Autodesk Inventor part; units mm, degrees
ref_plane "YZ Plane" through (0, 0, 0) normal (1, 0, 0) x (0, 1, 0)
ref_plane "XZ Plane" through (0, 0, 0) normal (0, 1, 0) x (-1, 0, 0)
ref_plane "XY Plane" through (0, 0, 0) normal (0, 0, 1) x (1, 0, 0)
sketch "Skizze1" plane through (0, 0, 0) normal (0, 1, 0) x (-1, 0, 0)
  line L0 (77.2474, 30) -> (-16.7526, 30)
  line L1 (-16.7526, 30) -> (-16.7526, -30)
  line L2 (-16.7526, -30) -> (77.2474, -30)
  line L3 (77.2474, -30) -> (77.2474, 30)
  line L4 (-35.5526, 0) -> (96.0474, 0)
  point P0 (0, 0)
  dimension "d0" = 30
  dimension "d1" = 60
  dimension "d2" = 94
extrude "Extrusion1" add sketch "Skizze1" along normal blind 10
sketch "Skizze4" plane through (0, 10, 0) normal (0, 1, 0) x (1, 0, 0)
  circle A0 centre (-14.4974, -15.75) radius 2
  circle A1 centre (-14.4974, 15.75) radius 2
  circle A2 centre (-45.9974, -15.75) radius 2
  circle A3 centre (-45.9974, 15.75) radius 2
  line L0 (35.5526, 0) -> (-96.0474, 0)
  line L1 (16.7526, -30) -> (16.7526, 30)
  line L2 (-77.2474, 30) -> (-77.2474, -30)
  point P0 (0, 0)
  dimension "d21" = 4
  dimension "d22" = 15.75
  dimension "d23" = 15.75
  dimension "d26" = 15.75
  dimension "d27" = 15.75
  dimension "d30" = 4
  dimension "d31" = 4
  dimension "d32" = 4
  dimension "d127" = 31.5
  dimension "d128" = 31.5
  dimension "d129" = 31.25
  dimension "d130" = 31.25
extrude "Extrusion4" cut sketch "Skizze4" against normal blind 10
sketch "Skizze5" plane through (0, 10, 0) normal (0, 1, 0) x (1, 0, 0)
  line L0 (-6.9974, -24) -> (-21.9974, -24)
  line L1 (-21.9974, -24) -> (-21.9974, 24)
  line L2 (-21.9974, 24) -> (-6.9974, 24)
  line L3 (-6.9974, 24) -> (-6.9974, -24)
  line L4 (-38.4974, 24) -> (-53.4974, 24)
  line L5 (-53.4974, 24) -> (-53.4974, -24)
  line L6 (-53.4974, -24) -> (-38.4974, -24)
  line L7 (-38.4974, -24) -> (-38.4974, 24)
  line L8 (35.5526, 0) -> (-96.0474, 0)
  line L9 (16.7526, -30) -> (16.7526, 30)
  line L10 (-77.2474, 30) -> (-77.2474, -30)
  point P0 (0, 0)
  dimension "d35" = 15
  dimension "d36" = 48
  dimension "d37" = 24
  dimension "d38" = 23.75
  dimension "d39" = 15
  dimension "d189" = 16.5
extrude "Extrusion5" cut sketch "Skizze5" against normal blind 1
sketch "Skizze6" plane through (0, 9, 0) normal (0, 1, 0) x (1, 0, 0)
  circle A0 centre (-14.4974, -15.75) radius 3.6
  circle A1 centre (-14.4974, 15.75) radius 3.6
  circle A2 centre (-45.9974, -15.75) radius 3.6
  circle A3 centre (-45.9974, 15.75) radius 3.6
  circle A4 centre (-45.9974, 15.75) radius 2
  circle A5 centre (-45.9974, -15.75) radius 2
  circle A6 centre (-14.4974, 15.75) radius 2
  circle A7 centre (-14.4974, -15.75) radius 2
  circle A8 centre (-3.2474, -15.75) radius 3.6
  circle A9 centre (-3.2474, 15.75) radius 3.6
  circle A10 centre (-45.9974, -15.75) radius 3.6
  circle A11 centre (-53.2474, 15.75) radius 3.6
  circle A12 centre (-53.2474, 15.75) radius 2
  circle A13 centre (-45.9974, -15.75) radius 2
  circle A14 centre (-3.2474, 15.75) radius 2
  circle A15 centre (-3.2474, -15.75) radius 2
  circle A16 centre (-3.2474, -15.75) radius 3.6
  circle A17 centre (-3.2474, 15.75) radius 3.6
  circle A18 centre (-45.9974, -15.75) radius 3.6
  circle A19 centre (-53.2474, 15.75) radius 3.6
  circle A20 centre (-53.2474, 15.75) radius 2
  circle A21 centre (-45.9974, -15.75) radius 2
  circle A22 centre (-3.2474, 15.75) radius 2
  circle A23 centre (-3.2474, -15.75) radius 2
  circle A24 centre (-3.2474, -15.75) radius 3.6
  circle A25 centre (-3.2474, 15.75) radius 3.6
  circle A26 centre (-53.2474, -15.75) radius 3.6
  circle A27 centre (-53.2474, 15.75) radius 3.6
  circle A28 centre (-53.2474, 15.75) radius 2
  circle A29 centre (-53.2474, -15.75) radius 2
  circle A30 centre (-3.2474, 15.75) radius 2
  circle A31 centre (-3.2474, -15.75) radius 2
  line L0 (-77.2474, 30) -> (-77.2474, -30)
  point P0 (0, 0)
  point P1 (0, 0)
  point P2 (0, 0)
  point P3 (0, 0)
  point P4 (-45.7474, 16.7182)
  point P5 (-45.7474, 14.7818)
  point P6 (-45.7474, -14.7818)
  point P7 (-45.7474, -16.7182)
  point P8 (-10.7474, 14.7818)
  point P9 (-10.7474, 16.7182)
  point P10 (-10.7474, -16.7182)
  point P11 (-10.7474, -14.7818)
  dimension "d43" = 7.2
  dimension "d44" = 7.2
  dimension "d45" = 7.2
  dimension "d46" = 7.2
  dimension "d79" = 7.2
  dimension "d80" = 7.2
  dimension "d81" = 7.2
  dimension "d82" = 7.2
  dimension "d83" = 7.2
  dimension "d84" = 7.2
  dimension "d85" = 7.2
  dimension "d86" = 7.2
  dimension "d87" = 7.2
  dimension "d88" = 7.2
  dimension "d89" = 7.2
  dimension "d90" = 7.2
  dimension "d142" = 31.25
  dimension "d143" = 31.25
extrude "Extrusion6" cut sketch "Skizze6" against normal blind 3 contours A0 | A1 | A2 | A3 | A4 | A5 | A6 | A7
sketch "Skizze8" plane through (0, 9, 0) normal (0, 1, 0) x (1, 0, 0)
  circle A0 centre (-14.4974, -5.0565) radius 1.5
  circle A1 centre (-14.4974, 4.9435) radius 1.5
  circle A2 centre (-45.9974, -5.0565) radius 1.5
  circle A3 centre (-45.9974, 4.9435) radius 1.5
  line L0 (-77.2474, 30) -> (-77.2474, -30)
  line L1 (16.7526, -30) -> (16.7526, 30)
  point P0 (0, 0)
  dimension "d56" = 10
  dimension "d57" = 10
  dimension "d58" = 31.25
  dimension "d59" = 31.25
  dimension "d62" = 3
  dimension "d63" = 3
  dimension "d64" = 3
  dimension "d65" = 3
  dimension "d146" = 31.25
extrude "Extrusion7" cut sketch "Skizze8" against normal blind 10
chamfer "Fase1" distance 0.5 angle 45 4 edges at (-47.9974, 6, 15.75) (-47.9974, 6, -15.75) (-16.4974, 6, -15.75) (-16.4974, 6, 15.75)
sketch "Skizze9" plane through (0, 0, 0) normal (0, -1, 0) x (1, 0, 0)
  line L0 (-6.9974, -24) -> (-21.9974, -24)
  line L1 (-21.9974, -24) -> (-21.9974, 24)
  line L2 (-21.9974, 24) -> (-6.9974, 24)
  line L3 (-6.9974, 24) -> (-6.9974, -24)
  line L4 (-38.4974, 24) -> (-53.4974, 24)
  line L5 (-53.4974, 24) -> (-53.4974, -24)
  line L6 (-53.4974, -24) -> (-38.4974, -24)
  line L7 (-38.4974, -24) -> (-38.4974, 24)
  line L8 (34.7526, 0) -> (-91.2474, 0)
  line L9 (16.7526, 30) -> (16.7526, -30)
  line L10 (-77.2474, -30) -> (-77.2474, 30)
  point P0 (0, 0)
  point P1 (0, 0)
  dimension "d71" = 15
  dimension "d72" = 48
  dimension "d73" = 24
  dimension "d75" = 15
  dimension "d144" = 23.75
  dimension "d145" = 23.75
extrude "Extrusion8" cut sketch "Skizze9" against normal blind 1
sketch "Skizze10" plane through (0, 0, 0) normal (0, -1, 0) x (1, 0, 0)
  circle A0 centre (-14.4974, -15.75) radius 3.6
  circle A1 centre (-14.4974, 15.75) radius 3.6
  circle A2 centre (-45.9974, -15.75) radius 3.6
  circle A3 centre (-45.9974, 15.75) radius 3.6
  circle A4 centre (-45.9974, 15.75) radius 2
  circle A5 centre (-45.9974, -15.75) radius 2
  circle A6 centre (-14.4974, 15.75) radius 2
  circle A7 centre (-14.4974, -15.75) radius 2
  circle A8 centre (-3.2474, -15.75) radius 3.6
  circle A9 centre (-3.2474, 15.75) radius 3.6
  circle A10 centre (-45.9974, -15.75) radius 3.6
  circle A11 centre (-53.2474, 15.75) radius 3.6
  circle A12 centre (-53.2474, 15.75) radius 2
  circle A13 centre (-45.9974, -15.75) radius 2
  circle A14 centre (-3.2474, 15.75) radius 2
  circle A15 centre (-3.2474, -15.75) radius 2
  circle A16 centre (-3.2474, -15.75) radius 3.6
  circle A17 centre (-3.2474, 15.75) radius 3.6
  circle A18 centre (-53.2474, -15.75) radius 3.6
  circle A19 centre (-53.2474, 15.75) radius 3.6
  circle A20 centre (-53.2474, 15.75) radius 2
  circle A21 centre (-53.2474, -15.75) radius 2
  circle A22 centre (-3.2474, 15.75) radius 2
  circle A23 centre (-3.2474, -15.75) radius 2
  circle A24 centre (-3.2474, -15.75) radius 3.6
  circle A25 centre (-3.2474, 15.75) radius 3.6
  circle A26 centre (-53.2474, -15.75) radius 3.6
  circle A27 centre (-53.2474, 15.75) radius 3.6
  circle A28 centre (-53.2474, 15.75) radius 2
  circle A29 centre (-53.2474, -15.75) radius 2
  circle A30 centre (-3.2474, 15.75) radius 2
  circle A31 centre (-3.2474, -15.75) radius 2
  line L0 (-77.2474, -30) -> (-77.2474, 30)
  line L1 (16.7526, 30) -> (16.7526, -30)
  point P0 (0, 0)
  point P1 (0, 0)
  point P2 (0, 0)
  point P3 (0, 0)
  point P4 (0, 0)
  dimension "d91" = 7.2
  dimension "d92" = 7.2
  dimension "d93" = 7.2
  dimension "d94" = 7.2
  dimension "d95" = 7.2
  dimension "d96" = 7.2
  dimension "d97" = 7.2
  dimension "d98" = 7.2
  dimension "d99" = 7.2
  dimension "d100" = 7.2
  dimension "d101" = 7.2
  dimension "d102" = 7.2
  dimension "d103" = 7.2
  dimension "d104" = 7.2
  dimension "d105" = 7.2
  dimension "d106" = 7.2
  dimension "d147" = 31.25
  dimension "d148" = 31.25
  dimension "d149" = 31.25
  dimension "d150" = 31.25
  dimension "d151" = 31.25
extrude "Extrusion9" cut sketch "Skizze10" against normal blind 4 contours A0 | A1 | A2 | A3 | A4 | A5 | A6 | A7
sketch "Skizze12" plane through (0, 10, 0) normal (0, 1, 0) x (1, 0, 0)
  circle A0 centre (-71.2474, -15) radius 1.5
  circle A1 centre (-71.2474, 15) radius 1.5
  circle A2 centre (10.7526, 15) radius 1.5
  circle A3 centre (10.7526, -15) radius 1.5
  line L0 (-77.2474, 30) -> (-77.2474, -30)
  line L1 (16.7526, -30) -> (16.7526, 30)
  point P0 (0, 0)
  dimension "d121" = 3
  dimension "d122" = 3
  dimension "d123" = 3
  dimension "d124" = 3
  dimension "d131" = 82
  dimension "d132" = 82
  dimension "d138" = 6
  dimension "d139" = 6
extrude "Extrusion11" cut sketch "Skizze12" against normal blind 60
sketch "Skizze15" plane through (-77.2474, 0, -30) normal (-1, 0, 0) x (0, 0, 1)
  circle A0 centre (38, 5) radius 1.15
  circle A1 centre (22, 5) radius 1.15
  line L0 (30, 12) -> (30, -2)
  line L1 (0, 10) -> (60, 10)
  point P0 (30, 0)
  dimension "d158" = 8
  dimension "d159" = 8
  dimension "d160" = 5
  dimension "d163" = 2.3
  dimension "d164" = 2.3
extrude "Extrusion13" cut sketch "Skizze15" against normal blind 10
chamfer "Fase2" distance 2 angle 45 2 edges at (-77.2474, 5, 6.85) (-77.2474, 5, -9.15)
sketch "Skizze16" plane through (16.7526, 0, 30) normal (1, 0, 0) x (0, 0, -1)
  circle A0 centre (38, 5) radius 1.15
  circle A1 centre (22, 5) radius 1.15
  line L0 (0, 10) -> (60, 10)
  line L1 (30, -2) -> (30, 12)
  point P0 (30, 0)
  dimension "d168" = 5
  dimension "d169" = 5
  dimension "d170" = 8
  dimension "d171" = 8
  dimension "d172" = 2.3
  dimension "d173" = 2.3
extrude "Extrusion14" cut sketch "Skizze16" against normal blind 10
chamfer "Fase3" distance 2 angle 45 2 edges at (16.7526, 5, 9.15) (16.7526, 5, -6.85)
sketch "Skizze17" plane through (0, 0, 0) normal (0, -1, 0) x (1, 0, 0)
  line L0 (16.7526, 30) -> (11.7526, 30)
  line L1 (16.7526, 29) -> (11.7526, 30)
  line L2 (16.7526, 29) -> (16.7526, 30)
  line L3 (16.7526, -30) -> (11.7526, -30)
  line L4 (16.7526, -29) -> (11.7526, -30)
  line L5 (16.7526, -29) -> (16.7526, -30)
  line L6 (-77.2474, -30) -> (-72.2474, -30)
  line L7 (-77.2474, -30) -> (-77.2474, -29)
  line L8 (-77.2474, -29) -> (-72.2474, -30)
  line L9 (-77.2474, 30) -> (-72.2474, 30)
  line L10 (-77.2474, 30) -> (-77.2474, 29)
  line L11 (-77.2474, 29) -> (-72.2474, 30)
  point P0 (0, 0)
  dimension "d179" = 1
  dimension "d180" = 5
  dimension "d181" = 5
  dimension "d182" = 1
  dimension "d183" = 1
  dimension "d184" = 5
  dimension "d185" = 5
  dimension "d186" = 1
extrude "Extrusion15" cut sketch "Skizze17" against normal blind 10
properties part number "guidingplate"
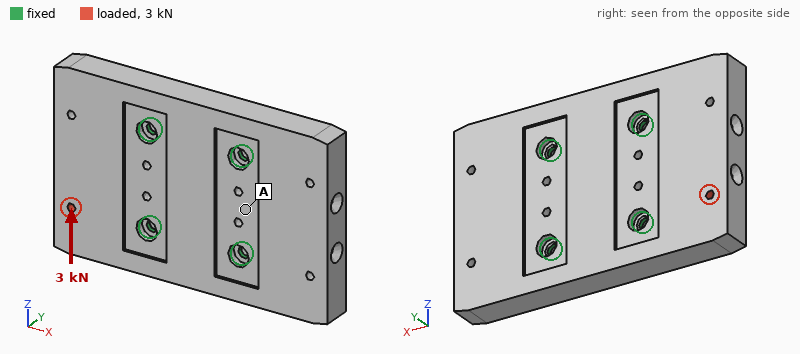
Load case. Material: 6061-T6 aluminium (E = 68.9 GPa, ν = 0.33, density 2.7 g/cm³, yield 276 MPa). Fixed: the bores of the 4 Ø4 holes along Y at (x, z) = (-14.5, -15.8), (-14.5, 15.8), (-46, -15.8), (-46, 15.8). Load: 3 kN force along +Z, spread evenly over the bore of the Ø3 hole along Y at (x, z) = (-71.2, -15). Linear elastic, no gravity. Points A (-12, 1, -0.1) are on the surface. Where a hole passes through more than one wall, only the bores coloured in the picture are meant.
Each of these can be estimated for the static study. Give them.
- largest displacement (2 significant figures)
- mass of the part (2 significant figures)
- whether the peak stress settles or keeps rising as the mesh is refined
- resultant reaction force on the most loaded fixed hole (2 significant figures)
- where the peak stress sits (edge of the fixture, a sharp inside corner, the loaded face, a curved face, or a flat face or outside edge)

22 µm
140 g
keeps rising
2.1 kN
edge of the fixture
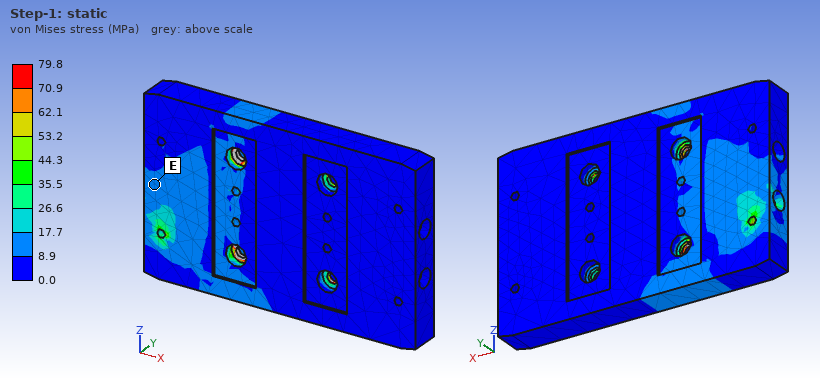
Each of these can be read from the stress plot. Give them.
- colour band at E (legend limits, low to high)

8.9 to 17.7 MPa
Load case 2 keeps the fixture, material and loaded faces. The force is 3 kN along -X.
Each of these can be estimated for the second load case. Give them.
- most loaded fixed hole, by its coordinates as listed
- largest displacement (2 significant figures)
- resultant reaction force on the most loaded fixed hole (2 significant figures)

(-46, -15.8)
11 µm
1.8 kN
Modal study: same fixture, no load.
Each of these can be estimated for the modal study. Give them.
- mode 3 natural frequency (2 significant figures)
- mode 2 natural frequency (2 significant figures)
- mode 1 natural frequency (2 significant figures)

6900 Hz
4000 Hz
3900 Hz
